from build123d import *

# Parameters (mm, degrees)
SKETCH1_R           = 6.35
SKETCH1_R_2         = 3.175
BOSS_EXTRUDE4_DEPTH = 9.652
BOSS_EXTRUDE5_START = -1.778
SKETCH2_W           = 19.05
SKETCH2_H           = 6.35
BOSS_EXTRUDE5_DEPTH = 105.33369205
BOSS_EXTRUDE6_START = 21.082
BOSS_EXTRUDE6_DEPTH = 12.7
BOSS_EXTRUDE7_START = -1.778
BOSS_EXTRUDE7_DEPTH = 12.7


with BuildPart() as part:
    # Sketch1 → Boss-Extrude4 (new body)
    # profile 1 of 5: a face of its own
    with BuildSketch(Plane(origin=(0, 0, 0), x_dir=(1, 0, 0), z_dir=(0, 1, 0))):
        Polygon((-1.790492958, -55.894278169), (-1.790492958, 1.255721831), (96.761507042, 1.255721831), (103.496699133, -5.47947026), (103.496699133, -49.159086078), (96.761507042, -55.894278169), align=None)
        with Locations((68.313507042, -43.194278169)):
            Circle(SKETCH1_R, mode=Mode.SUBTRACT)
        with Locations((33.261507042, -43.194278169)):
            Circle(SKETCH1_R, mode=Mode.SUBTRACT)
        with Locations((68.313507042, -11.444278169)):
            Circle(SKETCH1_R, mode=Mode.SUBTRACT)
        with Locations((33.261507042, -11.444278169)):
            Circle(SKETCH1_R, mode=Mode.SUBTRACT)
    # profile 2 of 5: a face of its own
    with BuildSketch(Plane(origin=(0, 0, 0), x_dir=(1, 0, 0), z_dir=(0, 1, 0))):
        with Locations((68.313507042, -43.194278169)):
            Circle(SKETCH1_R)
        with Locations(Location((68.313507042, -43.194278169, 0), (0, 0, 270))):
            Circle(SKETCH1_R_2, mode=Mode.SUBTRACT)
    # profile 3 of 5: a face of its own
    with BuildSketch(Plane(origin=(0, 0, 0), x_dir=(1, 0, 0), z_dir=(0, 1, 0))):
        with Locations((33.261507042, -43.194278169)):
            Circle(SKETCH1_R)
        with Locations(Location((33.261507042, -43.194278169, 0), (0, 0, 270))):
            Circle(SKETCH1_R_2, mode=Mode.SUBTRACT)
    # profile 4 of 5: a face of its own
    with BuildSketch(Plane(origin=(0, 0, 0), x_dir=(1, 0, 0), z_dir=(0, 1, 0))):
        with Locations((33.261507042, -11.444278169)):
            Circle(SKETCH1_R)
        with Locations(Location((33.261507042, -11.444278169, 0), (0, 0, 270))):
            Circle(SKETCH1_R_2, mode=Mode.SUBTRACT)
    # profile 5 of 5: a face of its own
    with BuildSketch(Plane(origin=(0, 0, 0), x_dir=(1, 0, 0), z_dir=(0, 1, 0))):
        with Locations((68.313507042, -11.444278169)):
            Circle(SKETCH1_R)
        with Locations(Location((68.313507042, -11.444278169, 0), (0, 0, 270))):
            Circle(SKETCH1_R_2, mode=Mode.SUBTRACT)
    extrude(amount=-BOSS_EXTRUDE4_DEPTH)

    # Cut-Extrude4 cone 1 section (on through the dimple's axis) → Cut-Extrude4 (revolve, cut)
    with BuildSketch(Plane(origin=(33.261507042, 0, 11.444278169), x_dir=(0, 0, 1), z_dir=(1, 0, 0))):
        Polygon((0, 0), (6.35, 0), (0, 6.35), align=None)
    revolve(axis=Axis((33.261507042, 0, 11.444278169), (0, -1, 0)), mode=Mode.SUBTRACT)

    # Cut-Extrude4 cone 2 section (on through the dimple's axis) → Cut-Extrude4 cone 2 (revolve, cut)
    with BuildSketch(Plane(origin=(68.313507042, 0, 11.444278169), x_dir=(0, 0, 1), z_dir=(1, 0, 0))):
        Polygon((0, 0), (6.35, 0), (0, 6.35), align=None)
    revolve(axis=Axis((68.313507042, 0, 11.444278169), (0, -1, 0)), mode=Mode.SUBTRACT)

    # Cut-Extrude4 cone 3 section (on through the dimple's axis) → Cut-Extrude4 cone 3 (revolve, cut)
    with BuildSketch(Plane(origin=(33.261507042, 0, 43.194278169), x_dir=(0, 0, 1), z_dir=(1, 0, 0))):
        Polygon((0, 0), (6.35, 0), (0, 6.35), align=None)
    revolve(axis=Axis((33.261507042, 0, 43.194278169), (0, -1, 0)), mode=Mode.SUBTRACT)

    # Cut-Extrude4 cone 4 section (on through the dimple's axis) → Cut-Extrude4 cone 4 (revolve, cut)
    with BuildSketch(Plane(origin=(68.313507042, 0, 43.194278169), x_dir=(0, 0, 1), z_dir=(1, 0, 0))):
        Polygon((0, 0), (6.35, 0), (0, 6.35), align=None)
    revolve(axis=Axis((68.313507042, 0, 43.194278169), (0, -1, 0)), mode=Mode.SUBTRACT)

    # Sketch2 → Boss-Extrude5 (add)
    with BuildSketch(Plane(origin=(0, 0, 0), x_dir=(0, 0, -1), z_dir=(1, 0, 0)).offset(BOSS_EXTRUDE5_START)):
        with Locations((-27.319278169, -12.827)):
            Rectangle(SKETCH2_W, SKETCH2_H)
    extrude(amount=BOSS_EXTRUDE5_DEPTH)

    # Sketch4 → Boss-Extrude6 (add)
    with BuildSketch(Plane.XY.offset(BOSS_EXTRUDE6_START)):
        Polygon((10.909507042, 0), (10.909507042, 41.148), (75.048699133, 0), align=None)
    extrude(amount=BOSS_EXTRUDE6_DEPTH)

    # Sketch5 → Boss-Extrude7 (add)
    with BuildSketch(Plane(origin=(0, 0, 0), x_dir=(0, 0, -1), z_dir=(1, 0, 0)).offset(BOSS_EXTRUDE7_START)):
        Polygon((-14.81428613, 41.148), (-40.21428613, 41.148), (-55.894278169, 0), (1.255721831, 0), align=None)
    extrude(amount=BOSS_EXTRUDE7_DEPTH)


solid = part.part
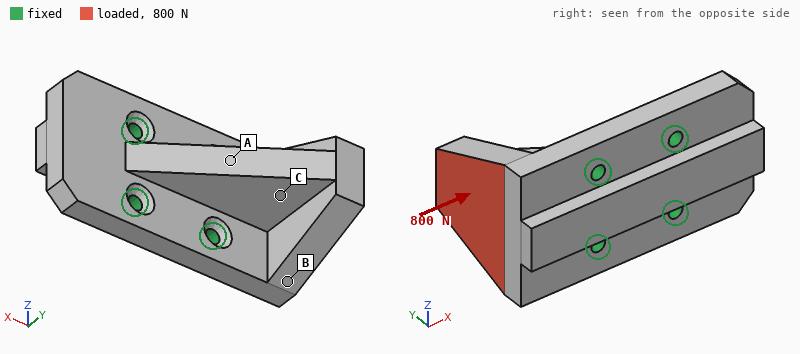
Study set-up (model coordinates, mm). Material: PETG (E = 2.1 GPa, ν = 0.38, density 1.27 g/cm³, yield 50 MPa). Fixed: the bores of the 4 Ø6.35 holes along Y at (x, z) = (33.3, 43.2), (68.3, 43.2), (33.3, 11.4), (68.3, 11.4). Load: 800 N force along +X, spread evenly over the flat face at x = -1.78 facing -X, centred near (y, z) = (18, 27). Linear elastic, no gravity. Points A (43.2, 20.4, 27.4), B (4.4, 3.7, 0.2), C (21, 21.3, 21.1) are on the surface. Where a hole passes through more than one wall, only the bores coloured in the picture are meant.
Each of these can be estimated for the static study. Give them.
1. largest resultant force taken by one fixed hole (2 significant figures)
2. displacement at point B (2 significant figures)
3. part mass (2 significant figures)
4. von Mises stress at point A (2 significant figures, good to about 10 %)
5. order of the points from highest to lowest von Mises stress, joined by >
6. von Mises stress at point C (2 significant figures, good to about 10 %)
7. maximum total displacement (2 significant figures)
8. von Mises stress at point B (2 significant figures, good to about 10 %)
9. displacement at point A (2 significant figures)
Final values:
310 N
0.16 mm
140 g
4.2 MPa
A > C > B
2.3 MPa
0.30 mm
1.00 MPa
0.10 mm
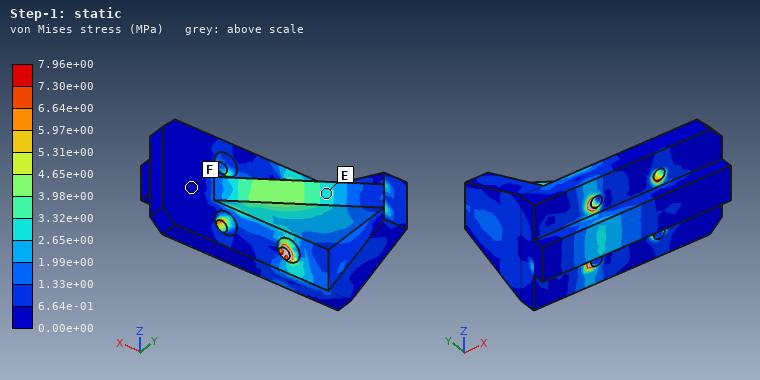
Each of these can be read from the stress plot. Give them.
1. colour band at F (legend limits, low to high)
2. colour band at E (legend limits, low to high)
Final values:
0.00e+00 to 6.64e-01 MPa
2.65e+00 to 3.32e+00 MPa
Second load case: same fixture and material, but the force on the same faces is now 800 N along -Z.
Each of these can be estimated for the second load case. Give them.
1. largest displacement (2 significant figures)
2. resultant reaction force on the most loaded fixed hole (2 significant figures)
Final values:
0.53 mm
930 N
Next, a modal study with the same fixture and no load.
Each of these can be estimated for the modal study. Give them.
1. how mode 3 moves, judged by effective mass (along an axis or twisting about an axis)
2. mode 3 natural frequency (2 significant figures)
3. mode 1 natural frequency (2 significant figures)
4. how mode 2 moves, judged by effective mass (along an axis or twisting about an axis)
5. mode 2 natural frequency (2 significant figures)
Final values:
along Y
1700 Hz
1100 Hz
along Z
1200 Hz
